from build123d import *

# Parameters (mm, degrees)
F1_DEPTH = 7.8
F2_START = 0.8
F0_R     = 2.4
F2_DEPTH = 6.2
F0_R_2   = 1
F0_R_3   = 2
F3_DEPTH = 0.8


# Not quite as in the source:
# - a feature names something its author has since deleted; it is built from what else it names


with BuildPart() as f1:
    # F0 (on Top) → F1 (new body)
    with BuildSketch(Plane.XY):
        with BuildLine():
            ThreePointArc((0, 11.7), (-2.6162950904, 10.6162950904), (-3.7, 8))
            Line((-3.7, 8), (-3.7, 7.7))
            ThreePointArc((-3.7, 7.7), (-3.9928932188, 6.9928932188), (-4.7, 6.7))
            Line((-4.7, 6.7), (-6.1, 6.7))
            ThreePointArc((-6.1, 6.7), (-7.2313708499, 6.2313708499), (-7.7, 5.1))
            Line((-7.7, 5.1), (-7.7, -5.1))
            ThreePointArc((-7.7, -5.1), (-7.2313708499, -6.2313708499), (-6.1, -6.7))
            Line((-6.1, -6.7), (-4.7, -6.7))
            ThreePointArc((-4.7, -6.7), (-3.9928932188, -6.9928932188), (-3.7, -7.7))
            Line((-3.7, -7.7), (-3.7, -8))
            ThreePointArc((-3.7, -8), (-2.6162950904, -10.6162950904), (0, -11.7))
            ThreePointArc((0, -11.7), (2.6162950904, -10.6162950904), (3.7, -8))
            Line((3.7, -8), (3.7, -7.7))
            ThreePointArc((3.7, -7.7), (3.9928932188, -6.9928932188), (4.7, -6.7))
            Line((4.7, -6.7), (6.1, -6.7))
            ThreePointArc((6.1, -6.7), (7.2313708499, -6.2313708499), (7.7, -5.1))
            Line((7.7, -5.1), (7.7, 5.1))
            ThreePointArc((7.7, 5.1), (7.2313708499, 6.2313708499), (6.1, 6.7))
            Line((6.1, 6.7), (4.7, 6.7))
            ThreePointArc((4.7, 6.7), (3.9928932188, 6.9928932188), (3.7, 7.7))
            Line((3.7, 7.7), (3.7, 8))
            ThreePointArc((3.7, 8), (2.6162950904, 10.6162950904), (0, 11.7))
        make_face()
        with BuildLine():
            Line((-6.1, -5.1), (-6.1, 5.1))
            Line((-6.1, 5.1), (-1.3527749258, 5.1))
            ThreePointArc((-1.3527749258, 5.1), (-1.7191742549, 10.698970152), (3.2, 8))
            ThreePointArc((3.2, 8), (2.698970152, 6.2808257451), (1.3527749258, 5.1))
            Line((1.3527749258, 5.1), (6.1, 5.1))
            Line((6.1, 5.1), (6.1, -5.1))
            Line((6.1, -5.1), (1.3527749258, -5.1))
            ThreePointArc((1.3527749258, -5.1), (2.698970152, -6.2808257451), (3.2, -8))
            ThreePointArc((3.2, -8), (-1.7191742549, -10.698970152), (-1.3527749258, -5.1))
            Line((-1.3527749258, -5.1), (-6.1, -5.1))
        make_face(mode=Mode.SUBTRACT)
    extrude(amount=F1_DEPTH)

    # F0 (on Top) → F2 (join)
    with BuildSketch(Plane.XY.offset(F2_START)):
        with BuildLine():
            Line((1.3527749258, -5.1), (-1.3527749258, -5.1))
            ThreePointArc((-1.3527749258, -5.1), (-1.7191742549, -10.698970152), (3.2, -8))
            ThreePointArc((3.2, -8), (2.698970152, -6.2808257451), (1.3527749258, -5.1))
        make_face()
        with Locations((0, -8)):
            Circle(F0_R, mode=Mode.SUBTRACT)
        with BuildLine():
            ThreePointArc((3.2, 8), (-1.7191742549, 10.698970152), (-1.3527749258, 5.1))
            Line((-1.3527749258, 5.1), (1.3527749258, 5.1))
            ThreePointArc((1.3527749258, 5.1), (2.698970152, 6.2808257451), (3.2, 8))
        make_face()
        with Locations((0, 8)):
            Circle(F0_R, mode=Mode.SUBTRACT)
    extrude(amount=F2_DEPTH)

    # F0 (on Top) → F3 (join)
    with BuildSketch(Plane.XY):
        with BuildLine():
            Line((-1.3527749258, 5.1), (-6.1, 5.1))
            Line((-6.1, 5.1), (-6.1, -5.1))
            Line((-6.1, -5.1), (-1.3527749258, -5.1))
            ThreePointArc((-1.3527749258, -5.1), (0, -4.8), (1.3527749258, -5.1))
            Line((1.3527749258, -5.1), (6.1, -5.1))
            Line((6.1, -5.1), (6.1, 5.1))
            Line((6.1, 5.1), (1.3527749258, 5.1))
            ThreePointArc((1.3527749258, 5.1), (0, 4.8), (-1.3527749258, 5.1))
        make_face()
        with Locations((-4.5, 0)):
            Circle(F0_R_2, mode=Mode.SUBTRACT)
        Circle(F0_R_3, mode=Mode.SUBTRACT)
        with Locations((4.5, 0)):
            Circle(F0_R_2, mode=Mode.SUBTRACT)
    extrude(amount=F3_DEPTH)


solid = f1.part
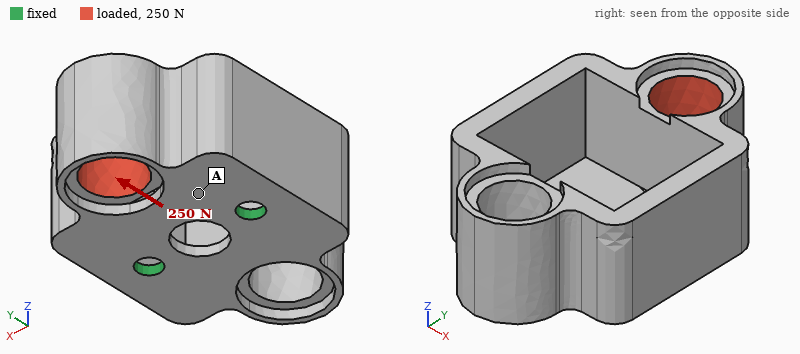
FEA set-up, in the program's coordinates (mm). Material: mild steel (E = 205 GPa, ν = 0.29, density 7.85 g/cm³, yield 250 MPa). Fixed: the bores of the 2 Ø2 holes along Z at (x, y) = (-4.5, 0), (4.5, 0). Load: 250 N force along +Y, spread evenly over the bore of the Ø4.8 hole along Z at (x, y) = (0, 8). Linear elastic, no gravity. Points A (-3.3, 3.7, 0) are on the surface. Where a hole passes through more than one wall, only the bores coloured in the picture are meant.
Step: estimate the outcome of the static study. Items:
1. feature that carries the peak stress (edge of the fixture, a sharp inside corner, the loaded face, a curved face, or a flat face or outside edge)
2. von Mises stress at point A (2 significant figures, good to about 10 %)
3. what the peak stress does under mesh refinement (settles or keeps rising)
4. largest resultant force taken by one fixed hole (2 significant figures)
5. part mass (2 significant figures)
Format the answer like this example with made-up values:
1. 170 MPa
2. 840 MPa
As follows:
1. edge of the fixture
2. 36 MPa
3. keeps rising
4. 130 N
5. 6.8 g
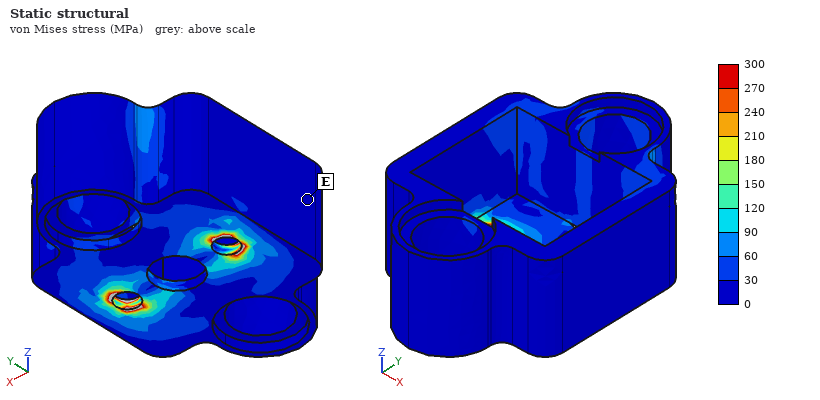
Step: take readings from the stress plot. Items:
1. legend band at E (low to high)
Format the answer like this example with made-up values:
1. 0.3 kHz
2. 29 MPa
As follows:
1. 0 to 30 MPa
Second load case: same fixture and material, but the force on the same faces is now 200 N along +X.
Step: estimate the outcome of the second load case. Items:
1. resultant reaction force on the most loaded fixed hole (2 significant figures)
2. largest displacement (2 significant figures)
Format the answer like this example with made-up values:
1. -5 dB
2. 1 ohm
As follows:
1. 180 N
2. 6.3 µm
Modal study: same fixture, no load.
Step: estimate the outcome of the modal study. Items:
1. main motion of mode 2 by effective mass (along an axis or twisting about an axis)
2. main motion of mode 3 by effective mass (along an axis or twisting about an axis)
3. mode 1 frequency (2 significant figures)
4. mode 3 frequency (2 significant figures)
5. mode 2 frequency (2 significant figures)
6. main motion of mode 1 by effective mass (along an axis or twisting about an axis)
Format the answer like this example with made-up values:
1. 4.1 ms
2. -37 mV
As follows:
1. along X
2. along Z
3. 4800 Hz
4. 21 kHz
5. 17 kHz
6. along Y
